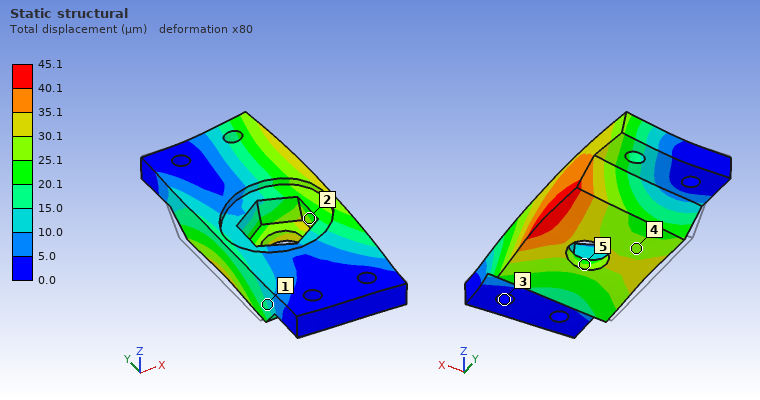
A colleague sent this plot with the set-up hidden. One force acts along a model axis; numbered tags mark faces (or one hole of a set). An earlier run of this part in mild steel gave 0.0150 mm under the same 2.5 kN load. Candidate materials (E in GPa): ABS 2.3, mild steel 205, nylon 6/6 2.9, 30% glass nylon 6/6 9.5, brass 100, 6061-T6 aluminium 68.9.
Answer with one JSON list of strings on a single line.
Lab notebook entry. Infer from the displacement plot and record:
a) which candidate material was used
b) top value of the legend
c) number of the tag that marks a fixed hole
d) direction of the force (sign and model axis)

["6061-T6 aluminium", "45.1 µm", "3", "+X"]
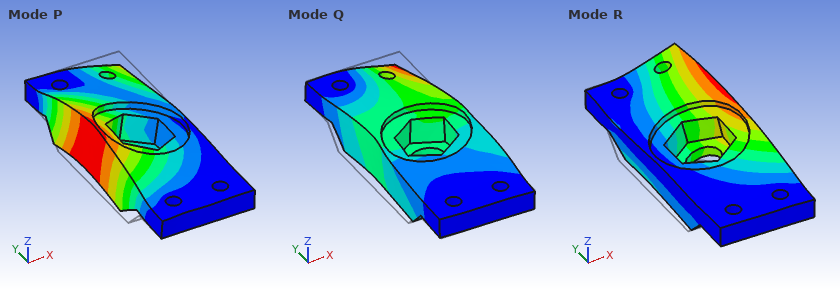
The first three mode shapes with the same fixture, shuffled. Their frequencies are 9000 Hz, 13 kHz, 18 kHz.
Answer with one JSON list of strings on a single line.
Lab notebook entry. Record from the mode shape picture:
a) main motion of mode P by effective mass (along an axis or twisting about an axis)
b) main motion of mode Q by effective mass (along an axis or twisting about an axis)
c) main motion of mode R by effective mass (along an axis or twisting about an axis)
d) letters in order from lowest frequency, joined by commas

["along Z", "along X", "along Z", "R, P, Q"]
